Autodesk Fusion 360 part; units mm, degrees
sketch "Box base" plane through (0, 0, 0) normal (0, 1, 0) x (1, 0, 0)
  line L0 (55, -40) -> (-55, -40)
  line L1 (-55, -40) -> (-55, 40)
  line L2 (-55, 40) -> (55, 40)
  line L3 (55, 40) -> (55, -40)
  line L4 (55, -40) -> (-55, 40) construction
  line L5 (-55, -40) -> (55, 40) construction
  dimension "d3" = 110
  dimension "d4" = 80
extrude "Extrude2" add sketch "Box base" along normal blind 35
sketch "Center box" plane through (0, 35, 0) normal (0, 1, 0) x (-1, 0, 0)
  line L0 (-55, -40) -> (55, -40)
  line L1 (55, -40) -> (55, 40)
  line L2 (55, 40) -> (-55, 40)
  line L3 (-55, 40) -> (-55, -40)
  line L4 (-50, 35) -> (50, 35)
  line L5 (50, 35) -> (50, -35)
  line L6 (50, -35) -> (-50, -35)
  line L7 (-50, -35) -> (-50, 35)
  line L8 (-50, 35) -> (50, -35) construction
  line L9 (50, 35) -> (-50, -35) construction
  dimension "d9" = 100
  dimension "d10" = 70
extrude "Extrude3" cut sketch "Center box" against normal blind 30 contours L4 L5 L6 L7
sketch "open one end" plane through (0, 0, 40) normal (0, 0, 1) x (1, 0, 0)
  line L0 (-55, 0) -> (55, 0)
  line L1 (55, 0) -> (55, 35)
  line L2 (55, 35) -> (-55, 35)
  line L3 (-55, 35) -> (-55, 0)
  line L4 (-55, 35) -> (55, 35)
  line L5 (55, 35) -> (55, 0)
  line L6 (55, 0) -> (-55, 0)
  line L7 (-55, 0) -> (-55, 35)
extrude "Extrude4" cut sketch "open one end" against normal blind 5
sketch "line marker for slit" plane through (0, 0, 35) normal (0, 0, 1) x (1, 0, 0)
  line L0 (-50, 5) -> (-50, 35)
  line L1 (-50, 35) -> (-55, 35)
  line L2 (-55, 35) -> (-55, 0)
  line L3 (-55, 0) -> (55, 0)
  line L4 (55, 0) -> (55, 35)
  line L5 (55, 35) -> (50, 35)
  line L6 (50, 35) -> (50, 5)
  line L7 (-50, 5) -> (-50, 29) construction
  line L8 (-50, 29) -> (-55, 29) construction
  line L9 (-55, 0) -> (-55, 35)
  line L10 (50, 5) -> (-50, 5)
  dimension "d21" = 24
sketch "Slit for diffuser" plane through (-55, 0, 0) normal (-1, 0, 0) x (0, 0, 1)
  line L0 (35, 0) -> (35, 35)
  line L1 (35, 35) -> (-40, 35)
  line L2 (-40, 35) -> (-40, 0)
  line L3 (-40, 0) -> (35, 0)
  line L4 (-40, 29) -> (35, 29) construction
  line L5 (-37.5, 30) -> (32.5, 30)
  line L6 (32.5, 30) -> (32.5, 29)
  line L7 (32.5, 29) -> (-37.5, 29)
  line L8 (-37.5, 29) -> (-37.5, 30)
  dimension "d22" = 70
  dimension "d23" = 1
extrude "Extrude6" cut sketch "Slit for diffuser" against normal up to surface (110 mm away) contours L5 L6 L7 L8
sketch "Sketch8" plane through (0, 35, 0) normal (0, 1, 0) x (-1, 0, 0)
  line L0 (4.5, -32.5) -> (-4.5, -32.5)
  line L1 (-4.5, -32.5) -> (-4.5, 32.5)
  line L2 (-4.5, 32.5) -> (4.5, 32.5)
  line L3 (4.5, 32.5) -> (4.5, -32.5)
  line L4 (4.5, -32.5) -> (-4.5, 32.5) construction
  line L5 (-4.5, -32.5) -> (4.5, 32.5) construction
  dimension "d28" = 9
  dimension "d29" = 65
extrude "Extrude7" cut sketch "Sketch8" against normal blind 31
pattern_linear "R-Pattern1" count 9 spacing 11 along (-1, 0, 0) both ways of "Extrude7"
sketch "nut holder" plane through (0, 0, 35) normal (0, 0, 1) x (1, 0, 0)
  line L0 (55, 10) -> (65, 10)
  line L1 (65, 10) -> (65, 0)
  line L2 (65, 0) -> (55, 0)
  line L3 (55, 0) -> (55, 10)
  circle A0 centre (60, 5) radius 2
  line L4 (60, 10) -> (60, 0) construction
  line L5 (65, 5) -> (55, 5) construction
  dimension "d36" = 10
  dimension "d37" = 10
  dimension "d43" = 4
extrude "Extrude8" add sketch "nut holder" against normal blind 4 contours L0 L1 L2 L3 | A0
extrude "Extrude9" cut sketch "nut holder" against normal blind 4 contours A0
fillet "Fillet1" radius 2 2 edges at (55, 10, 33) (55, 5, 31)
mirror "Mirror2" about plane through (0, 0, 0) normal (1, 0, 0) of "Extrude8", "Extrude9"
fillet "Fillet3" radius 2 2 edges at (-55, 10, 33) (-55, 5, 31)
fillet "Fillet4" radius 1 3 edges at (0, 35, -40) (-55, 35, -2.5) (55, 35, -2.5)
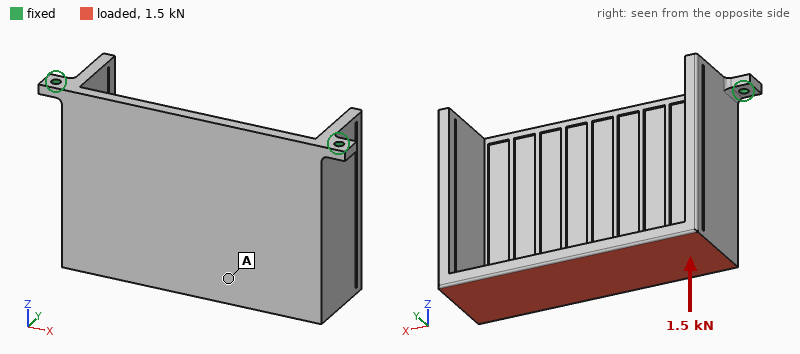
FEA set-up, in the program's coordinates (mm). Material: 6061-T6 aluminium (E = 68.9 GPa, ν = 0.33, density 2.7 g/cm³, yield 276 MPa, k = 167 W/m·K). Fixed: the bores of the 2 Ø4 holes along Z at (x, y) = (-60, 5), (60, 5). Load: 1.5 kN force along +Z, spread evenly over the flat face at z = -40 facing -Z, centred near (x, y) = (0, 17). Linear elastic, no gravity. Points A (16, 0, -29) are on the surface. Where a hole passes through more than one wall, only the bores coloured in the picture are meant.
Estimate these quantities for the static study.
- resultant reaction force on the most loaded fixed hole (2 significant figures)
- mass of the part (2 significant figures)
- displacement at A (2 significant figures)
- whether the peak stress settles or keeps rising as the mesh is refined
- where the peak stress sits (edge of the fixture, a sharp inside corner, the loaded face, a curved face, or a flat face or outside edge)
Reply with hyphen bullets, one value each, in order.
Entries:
- 770 N
- 200 g
- 0.49 mm
- keeps rising
- edge of the fixture
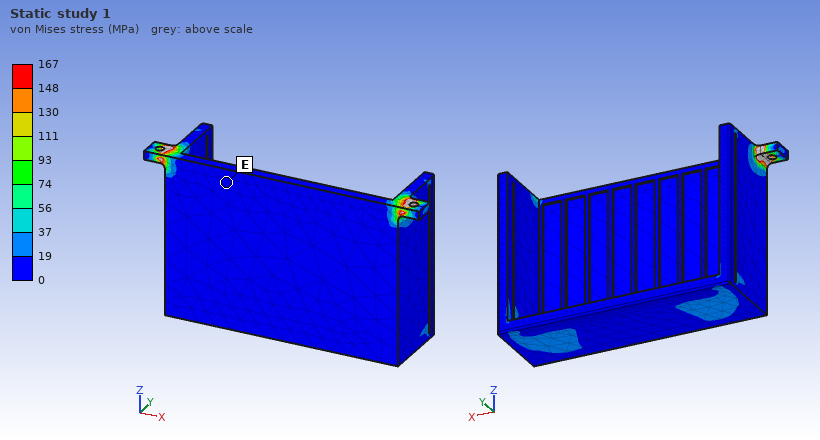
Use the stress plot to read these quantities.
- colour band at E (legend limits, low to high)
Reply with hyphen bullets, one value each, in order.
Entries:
- 0 to 19 MPa
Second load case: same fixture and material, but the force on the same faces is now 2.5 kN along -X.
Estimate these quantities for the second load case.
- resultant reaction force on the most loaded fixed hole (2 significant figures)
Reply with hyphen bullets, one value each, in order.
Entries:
- 2.0 kN
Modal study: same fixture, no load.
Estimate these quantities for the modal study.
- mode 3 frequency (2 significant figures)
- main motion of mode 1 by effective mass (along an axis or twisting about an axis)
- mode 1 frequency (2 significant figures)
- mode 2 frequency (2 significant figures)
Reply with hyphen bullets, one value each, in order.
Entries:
- 1900 Hz
- along Y
- 330 Hz
- 770 Hz
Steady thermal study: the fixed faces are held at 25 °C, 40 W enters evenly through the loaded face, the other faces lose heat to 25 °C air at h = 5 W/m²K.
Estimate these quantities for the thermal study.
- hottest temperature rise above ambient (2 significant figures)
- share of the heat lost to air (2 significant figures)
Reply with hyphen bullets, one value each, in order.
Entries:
- 48 K
- 14 %
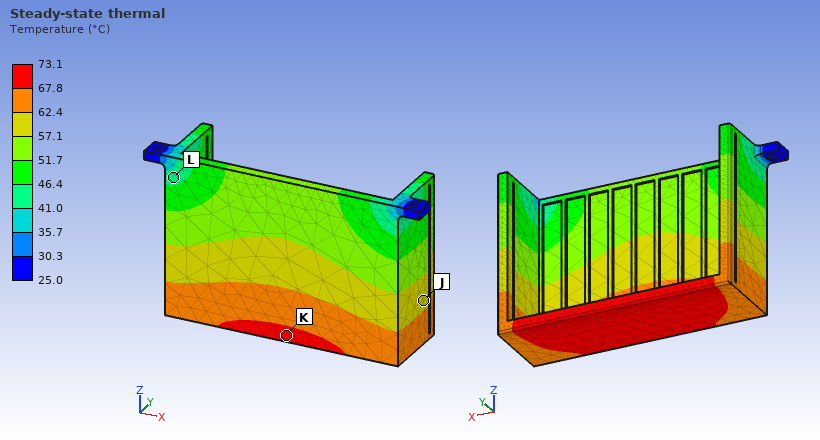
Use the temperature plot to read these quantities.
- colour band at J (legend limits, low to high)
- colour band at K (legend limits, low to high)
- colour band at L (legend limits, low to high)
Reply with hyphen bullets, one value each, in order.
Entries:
- 57.1 to 62.4 °C
- 67.8 to 73.1 °C
- 41.0 to 46.4 °C
